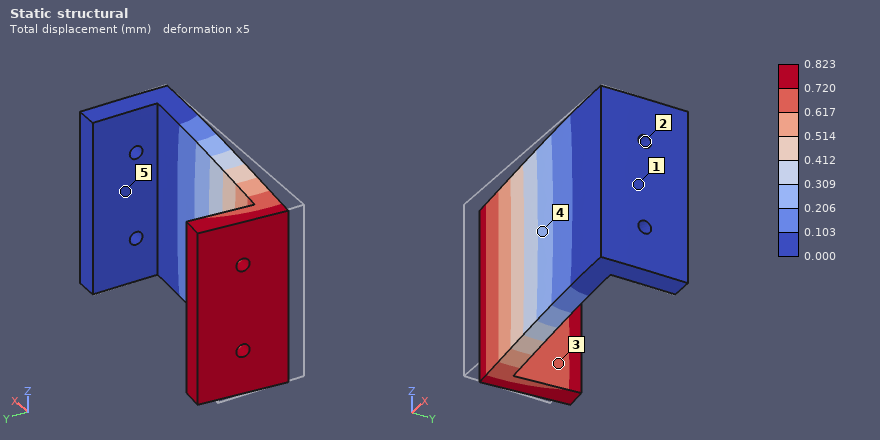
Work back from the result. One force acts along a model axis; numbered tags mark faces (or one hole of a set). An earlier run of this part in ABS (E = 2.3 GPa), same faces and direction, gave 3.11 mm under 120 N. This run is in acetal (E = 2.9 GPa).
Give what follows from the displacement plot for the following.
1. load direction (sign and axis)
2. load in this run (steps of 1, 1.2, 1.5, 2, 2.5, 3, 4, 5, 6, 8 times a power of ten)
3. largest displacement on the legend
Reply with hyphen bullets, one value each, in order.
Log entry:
- +Y
- 40 N
- 0.823 mm
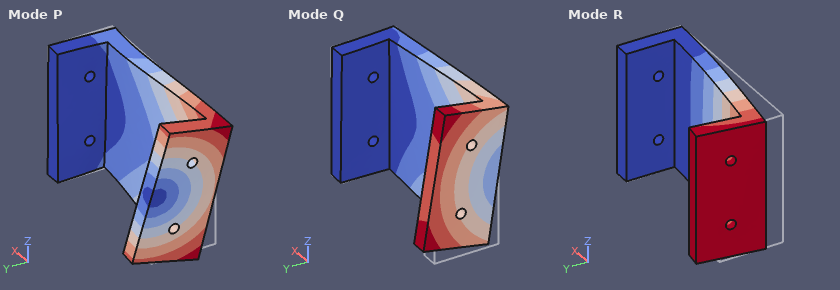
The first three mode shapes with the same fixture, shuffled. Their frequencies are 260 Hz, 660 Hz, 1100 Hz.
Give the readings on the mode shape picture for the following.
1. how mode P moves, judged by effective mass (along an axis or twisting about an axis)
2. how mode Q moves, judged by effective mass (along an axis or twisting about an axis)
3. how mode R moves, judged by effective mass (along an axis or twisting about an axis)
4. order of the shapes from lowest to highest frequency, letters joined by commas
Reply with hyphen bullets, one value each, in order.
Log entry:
- along Z
- along Z
- along Y
- R, Q, P
